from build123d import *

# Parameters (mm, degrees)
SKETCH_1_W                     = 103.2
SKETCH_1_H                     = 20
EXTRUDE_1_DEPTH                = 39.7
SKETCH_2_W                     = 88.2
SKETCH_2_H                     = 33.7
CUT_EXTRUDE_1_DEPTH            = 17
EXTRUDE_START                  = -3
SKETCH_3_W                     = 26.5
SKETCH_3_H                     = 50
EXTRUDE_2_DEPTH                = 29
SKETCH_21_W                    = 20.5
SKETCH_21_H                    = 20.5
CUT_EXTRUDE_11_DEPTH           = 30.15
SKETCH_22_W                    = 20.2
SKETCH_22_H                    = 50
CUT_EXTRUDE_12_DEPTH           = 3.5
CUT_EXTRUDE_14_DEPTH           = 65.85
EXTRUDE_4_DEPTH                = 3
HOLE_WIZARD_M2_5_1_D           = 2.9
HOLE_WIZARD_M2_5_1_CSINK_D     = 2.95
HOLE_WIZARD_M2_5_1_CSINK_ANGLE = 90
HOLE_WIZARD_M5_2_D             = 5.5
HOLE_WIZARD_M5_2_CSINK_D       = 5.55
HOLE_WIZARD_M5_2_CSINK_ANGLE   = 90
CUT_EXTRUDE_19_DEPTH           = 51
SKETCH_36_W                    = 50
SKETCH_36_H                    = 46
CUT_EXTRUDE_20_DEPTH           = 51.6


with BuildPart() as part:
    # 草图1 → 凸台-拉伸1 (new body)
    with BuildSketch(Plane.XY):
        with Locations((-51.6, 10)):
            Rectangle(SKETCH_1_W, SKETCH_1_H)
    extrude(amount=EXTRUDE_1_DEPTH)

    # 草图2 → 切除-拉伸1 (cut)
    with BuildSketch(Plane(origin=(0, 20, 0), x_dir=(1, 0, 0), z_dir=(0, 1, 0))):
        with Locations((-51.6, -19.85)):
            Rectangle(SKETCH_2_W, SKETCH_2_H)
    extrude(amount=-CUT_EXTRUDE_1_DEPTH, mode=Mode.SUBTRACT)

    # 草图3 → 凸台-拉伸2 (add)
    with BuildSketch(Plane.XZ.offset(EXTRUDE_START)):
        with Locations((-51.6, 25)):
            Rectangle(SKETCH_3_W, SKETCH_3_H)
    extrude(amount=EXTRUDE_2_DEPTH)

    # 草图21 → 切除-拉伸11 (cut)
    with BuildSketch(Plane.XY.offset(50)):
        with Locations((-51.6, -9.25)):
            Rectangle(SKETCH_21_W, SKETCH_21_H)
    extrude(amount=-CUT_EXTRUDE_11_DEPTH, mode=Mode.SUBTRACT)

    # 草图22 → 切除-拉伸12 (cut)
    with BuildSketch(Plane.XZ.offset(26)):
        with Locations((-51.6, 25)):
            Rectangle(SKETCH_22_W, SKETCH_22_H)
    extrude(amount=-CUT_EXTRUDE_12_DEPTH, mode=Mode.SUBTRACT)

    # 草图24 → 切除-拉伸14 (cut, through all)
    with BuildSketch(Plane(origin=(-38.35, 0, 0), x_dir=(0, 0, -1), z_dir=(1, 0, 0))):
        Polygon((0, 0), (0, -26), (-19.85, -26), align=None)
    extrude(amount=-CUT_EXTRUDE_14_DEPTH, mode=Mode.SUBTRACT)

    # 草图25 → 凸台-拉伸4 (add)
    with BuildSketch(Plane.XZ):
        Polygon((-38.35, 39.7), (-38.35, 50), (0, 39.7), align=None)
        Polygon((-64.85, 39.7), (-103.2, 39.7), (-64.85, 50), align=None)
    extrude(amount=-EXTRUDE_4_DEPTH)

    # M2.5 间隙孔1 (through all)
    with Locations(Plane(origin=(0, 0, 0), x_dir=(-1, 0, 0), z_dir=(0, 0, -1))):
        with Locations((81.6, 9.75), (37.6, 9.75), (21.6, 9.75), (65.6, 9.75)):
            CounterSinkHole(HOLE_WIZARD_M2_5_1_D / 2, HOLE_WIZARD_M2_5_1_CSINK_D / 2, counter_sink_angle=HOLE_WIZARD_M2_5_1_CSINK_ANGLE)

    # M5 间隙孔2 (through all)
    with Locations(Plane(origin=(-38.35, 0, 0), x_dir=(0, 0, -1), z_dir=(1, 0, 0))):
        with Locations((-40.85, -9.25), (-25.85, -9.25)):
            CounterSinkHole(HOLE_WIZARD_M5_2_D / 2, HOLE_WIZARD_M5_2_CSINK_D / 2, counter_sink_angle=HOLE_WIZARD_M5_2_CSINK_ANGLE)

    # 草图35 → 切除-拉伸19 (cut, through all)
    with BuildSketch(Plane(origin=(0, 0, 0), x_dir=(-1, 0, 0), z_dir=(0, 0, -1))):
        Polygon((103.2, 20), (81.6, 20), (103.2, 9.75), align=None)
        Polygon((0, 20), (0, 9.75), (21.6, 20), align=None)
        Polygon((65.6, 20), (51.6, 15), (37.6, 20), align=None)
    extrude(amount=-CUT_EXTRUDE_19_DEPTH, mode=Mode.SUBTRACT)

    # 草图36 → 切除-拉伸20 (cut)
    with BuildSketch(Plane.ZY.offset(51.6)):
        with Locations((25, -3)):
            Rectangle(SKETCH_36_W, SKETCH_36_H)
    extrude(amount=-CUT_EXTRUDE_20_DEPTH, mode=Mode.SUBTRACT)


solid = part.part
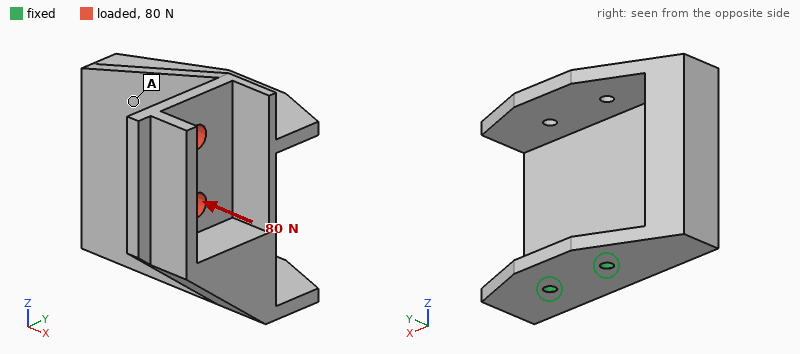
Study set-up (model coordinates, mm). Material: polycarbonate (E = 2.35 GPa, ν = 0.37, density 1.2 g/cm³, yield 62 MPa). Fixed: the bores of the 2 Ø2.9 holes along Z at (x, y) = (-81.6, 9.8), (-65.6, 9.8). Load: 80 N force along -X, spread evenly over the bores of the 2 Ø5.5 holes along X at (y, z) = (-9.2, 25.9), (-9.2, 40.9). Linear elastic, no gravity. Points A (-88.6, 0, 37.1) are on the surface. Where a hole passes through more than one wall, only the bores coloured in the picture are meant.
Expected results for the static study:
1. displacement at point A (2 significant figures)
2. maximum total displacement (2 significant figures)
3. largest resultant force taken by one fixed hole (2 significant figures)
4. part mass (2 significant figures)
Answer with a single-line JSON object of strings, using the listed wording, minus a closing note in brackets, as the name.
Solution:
{"displacement at point A": "0.53 mm", "maximum total displacement": "0.98 mm", "largest resultant force taken by one fixed hole": "150 N", "part mass": "24 g"}
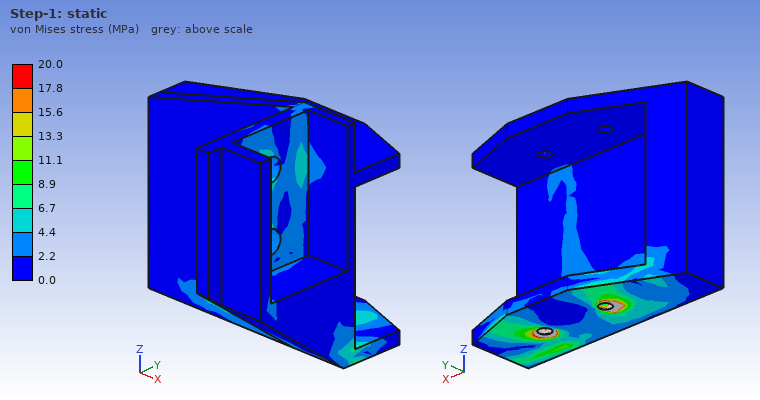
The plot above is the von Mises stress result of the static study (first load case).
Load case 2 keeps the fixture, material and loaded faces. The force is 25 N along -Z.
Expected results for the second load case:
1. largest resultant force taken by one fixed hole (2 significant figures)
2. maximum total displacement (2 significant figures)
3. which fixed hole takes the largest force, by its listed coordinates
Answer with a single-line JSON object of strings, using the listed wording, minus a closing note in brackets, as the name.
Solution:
{"largest resultant force taken by one fixed hole": "24 N", "maximum total displacement": "0.95 mm", "which fixed hole takes the largest force, by its listed coordinates": "(-65.6, 9.8)"}
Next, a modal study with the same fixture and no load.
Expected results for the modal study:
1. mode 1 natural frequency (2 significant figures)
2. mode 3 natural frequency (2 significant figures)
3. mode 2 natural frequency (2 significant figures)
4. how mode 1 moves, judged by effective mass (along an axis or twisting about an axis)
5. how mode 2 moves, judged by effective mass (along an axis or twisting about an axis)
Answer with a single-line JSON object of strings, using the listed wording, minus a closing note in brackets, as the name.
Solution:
{"mode 1 natural frequency": "190 Hz", "mode 3 natural frequency": "680 Hz", "mode 2 natural frequency": "450 Hz", "how mode 1 moves, judged by effective mass": "along Y", "how mode 2 moves, judged by effective mass": "along X"}
